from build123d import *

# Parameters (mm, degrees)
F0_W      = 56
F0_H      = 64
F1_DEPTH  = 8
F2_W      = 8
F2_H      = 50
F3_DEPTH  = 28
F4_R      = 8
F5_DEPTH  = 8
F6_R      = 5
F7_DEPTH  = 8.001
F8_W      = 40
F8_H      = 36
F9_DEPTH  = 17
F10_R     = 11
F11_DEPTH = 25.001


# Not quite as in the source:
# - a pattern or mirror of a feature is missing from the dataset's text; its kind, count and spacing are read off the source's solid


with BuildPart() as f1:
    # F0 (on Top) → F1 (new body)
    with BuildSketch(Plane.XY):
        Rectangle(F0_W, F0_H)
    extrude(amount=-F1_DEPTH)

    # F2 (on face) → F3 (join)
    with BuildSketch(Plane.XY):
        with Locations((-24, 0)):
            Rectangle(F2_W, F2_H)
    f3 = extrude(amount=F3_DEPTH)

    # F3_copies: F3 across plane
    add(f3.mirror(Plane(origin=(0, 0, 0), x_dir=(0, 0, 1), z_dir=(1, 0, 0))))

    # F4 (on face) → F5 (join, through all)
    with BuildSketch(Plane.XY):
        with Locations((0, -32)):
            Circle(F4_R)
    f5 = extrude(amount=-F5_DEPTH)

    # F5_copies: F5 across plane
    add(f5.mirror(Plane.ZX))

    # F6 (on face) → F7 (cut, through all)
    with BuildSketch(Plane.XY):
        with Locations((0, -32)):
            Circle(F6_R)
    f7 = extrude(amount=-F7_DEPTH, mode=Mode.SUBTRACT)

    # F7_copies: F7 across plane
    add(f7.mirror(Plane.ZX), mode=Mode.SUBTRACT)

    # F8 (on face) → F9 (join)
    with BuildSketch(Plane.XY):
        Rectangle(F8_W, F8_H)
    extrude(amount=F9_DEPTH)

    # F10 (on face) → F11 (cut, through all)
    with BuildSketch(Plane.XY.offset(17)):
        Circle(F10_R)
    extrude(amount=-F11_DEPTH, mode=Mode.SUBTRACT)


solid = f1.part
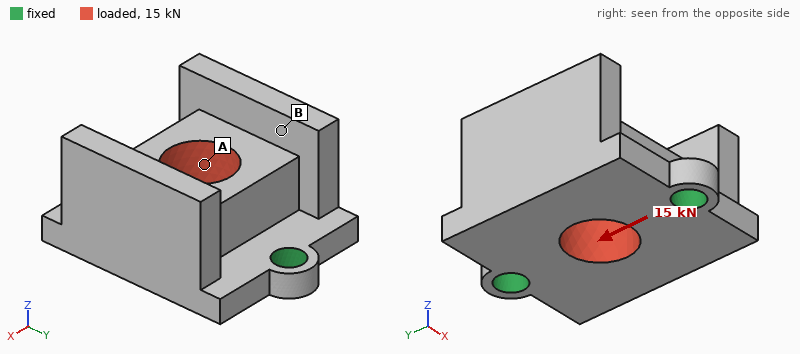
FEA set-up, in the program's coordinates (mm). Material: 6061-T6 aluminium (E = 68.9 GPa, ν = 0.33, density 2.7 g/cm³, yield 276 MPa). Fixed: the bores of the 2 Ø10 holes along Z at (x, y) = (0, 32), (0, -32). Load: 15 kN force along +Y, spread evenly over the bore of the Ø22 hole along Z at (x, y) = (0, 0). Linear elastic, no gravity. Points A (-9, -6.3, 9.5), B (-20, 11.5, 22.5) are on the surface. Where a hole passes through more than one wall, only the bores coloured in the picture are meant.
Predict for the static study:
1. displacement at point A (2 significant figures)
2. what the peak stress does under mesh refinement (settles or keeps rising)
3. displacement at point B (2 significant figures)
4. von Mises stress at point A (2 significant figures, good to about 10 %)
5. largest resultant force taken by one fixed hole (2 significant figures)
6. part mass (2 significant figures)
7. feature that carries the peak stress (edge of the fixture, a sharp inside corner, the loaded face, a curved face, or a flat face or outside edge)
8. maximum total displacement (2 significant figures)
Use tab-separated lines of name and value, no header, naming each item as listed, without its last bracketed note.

displacement at point A	21 µm
what the peak stress does under mesh refinement	keeps rising
displacement at point B	26 µm
von Mises stress at point A	24 MPa
largest resultant force taken by one fixed hole	7.9 kN
part mass	180 g
feature that carries the peak stress	edge of the fixture
maximum total displacement	31 µm
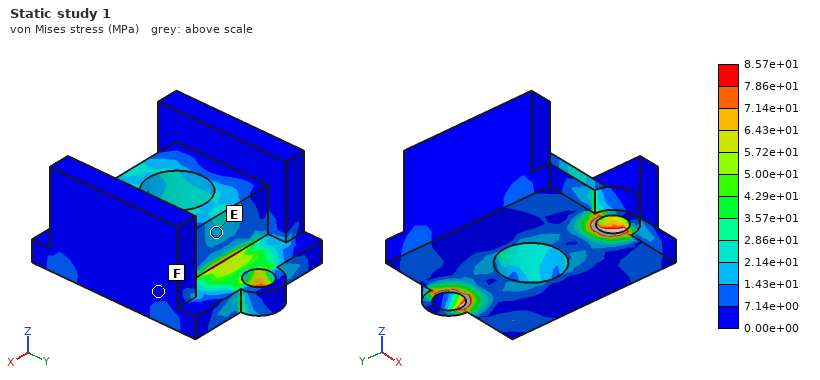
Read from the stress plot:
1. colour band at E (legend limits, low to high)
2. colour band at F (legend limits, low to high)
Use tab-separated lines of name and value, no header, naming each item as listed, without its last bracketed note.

colour band at E	1.43e+01 to 2.14e+01 MPa
colour band at F	0.00e+00 to 7.14e+00 MPa
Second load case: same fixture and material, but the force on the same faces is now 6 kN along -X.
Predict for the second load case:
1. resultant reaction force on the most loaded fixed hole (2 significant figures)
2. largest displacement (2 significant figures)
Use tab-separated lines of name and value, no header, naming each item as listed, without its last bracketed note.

resultant reaction force on the most loaded fixed hole	3.0 kN
largest displacement	84 µm
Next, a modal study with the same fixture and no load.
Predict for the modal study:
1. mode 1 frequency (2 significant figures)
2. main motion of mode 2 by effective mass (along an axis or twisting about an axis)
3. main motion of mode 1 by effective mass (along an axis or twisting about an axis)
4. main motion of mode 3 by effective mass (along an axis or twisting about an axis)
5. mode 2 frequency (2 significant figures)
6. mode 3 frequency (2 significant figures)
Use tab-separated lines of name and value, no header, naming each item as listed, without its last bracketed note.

mode 1 frequency	2800 Hz
main motion of mode 2 by effective mass	along Z
main motion of mode 1 by effective mass	along X
main motion of mode 3 by effective mass	along Y
mode 2 frequency	6500 Hz
mode 3 frequency	8200 Hz
